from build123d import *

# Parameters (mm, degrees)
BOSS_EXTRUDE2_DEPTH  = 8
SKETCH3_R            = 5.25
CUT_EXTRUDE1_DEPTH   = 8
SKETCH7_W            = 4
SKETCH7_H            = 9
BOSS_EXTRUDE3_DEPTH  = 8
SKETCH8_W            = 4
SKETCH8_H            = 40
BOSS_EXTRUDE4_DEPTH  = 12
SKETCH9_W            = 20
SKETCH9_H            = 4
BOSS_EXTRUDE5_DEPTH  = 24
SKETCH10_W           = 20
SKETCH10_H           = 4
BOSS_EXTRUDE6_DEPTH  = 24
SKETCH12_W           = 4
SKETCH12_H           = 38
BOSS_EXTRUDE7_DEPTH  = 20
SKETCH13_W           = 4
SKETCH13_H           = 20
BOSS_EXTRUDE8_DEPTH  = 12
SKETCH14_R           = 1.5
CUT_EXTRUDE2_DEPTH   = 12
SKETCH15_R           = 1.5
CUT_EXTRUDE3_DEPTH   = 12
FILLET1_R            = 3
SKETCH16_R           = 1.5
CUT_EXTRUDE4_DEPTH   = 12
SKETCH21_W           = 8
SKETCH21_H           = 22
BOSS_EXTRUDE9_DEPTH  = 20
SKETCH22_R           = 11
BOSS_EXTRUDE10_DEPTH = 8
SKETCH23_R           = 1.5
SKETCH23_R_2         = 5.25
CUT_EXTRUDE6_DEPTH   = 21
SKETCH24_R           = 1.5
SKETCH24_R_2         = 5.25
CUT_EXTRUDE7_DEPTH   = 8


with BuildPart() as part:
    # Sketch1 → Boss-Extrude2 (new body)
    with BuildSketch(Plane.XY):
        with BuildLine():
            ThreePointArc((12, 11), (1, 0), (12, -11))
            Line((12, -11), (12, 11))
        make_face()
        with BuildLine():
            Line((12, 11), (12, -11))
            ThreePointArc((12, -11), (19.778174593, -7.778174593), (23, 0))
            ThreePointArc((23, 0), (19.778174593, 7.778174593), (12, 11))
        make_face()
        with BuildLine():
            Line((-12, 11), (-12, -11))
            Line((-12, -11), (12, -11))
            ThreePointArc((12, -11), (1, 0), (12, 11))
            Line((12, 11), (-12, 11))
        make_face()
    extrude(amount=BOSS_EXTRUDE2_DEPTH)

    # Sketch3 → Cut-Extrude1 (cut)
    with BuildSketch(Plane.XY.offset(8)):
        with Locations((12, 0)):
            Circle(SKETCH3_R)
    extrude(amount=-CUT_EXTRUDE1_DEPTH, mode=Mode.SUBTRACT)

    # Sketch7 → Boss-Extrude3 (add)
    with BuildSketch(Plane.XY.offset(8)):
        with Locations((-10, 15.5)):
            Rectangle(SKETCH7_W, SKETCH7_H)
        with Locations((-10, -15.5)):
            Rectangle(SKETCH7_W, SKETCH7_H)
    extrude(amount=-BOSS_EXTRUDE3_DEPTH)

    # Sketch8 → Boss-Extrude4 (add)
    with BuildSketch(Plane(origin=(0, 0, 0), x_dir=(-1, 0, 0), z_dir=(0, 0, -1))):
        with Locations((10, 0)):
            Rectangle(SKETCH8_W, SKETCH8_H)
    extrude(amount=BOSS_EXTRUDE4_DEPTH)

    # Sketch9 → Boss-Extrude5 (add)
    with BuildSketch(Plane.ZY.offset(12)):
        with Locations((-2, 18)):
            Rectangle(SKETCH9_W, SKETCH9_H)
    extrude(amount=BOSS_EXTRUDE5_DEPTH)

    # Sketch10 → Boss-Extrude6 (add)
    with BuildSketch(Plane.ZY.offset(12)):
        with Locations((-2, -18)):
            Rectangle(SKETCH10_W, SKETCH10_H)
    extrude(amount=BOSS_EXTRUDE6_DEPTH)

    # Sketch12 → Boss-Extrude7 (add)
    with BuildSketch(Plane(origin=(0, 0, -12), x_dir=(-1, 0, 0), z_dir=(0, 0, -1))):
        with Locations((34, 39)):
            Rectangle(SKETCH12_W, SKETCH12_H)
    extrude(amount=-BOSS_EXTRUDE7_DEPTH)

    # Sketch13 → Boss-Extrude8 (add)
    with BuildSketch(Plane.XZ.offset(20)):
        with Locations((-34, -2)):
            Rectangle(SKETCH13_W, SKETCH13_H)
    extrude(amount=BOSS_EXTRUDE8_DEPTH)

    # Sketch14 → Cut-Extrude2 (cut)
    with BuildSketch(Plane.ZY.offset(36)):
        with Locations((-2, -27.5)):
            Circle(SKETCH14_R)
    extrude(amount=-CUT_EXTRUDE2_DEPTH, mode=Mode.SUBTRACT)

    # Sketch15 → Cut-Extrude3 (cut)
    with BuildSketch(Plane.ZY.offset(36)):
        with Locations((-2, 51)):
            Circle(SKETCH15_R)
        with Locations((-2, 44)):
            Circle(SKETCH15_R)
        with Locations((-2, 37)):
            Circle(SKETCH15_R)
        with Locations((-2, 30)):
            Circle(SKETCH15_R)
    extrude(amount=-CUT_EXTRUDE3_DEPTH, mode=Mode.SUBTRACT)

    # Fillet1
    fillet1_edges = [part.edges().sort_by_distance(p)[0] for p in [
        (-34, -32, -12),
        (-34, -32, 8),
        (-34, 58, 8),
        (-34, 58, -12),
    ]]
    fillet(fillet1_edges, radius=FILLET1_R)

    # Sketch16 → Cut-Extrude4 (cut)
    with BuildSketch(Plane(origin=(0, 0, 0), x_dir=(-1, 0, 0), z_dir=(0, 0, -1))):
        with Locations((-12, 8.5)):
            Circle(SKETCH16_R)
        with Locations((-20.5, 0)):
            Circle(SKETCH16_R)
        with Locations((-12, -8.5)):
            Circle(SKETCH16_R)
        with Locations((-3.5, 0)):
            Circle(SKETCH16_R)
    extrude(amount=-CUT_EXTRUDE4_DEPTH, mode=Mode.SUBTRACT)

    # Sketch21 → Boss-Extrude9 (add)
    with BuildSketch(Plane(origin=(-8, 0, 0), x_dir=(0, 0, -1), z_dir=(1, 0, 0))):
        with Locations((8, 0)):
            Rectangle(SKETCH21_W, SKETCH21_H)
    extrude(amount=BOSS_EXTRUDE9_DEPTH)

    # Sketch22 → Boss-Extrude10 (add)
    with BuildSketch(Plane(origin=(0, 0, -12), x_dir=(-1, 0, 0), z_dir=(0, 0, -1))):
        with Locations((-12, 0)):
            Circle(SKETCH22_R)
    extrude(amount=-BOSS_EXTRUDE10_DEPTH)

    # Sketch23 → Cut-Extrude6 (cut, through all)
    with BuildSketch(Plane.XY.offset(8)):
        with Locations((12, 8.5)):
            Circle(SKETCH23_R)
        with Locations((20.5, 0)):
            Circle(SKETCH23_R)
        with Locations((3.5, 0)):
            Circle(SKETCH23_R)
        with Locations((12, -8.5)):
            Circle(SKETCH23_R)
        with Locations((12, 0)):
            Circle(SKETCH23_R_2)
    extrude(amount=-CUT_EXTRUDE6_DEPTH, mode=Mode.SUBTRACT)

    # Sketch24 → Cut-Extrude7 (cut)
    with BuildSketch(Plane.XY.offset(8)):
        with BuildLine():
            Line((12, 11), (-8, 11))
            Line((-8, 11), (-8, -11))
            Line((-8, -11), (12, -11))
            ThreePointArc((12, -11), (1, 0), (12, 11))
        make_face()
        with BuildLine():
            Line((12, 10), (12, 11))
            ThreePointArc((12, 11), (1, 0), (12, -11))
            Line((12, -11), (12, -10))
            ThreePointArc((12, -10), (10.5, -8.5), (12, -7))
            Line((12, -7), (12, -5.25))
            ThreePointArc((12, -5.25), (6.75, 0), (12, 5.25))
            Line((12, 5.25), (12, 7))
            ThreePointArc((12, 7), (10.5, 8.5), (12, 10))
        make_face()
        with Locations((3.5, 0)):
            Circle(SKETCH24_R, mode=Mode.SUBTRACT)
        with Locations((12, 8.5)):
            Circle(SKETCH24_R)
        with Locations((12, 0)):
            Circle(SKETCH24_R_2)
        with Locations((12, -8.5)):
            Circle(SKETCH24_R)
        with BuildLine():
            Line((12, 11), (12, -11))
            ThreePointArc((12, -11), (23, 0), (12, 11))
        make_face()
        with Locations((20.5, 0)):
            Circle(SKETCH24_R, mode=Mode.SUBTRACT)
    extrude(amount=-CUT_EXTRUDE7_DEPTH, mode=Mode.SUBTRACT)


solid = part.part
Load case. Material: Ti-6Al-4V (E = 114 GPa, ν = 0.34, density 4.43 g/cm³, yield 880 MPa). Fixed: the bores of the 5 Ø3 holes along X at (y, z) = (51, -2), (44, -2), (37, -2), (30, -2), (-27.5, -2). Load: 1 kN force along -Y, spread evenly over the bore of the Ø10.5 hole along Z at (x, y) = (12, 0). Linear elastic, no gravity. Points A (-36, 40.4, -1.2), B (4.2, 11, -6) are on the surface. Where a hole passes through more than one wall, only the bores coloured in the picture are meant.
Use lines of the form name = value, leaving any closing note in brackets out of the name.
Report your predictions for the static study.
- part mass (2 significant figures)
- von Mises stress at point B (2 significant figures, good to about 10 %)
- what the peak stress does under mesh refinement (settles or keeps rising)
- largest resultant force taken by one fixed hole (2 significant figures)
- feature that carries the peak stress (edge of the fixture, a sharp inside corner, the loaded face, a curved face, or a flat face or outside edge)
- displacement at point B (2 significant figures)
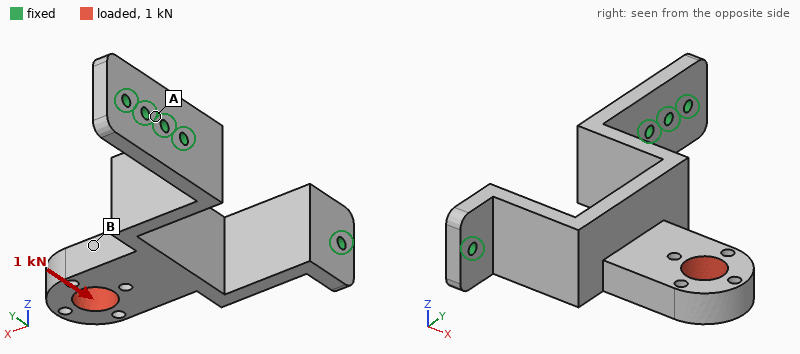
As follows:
part mass = 66 g
von Mises stress at point B = 23 MPa
what the peak stress does under mesh refinement = keeps rising
largest resultant force taken by one fixed hole = 1.1 kN
feature that carries the peak stress = edge of the fixture
displacement at point B = 0.076 mm
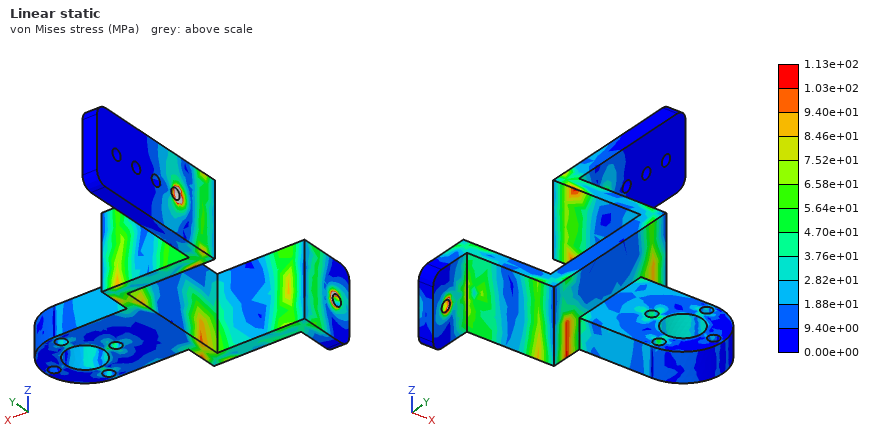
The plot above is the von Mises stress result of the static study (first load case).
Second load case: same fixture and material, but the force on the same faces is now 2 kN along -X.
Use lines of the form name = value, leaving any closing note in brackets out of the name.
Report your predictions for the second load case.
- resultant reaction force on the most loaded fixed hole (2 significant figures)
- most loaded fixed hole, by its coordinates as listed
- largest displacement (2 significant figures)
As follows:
resultant reaction force on the most loaded fixed hole = 1.3 kN
most loaded fixed hole, by its coordinates as listed = (30, -2)
largest displacement = 0.26 mm
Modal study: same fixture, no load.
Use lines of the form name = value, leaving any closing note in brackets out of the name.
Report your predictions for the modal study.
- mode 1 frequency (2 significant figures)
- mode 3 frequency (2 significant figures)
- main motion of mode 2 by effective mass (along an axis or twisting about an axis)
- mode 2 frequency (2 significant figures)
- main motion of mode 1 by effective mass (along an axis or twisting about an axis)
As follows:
mode 1 frequency = 1300 Hz
mode 3 frequency = 5000 Hz
main motion of mode 2 by effective mass = along Y
mode 2 frequency = 3000 Hz
main motion of mode 1 by effective mass = along Z
